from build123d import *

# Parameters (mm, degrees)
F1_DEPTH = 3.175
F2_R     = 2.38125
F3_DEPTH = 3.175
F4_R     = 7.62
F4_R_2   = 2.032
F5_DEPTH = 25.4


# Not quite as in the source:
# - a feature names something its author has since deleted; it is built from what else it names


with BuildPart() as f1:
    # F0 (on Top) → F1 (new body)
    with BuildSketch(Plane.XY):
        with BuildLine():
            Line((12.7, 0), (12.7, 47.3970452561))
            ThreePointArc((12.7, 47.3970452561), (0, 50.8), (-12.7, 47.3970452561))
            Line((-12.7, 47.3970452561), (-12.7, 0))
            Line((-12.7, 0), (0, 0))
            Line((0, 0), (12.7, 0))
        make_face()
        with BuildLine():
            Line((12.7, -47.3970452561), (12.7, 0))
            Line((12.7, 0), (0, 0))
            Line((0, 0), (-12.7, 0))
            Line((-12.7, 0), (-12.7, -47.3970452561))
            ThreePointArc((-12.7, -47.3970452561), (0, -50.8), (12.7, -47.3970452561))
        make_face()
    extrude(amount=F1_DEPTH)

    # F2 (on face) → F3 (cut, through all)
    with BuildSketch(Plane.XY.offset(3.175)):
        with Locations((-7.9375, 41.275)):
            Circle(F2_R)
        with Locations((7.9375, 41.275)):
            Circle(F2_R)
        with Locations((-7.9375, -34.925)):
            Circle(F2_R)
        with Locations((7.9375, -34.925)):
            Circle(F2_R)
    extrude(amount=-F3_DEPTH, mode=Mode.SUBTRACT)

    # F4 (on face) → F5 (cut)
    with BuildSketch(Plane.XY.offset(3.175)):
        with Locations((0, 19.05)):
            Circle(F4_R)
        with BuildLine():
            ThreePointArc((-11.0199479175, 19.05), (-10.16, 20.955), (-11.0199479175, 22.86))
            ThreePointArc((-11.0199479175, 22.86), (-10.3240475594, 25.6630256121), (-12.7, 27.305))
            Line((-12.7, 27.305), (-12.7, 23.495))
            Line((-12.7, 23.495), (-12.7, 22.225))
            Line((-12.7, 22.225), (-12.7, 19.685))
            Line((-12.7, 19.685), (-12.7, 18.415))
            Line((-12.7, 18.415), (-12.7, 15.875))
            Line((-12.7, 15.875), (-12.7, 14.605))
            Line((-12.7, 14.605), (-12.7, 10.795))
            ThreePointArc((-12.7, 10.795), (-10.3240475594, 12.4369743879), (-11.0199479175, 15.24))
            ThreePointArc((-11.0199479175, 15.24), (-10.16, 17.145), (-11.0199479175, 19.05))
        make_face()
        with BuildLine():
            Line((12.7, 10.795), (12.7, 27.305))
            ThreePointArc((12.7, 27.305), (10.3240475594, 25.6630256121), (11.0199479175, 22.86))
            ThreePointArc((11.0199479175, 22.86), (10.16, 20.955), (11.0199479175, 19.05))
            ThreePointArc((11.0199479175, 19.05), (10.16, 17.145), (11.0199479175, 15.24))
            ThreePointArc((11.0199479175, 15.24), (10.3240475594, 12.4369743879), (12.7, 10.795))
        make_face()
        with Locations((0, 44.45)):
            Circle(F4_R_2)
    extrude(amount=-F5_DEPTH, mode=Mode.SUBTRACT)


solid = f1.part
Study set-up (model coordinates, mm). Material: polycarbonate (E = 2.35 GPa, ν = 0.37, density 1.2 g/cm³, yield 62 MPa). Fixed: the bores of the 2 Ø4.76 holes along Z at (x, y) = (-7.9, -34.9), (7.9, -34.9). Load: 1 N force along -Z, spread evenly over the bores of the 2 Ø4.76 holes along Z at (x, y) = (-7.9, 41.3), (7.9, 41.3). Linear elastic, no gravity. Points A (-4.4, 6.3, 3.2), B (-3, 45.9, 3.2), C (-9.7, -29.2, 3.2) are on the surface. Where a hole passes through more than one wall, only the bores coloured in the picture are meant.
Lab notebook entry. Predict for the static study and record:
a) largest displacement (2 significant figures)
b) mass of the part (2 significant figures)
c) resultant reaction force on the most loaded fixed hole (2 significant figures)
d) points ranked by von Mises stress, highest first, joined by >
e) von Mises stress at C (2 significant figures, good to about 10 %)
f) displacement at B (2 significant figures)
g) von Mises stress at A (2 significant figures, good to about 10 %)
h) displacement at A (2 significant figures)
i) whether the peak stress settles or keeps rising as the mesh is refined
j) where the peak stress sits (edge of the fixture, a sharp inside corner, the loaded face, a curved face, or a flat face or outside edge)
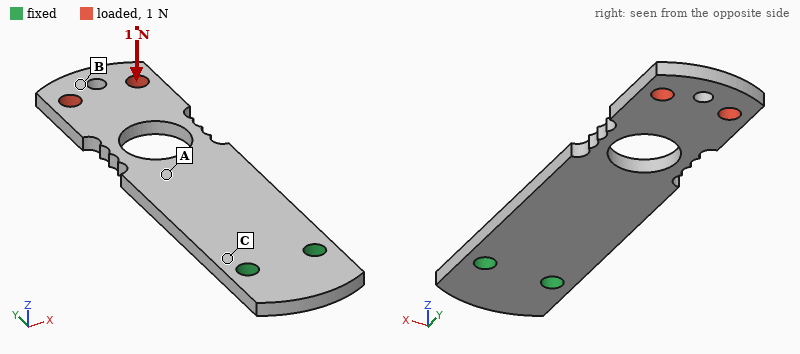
1.2 mm
8.3 g
0.50 N
C > A > B
1.6 MPa
1.1 mm
0.83 MPa
0.30 mm
keeps rising
edge of the fixture
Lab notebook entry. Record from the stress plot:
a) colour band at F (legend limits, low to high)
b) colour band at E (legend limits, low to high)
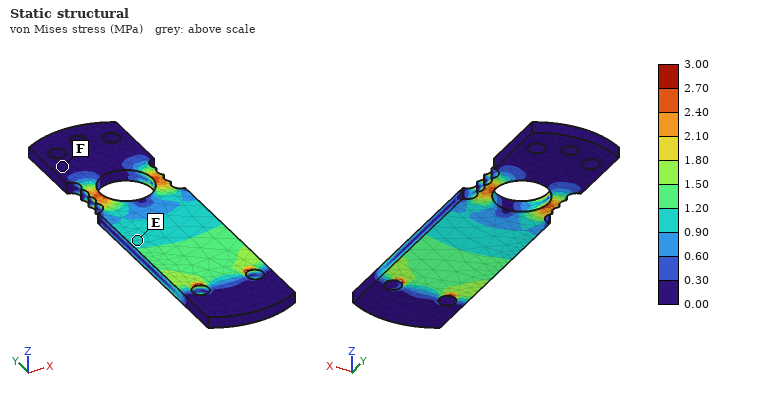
0.00 to 0.30 MPa
0.90 to 1.20 MPa
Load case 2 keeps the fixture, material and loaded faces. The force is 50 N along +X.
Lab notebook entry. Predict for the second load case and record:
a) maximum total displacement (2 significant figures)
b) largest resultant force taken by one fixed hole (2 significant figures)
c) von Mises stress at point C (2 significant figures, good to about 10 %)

1.2 mm
210 N
8.4 MPa
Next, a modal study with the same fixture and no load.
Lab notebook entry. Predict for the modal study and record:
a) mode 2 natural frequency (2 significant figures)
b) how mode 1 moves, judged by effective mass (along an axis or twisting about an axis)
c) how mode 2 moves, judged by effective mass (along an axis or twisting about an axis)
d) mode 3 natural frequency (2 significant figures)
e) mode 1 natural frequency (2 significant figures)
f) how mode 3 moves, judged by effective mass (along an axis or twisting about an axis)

550 Hz
along Z
along Z
650 Hz
110 Hz
twisting about Y
